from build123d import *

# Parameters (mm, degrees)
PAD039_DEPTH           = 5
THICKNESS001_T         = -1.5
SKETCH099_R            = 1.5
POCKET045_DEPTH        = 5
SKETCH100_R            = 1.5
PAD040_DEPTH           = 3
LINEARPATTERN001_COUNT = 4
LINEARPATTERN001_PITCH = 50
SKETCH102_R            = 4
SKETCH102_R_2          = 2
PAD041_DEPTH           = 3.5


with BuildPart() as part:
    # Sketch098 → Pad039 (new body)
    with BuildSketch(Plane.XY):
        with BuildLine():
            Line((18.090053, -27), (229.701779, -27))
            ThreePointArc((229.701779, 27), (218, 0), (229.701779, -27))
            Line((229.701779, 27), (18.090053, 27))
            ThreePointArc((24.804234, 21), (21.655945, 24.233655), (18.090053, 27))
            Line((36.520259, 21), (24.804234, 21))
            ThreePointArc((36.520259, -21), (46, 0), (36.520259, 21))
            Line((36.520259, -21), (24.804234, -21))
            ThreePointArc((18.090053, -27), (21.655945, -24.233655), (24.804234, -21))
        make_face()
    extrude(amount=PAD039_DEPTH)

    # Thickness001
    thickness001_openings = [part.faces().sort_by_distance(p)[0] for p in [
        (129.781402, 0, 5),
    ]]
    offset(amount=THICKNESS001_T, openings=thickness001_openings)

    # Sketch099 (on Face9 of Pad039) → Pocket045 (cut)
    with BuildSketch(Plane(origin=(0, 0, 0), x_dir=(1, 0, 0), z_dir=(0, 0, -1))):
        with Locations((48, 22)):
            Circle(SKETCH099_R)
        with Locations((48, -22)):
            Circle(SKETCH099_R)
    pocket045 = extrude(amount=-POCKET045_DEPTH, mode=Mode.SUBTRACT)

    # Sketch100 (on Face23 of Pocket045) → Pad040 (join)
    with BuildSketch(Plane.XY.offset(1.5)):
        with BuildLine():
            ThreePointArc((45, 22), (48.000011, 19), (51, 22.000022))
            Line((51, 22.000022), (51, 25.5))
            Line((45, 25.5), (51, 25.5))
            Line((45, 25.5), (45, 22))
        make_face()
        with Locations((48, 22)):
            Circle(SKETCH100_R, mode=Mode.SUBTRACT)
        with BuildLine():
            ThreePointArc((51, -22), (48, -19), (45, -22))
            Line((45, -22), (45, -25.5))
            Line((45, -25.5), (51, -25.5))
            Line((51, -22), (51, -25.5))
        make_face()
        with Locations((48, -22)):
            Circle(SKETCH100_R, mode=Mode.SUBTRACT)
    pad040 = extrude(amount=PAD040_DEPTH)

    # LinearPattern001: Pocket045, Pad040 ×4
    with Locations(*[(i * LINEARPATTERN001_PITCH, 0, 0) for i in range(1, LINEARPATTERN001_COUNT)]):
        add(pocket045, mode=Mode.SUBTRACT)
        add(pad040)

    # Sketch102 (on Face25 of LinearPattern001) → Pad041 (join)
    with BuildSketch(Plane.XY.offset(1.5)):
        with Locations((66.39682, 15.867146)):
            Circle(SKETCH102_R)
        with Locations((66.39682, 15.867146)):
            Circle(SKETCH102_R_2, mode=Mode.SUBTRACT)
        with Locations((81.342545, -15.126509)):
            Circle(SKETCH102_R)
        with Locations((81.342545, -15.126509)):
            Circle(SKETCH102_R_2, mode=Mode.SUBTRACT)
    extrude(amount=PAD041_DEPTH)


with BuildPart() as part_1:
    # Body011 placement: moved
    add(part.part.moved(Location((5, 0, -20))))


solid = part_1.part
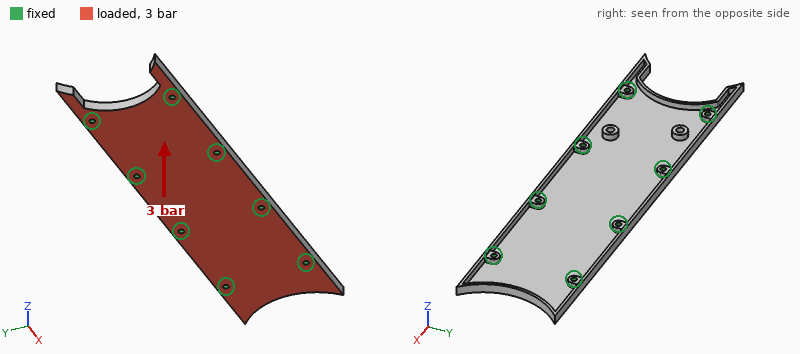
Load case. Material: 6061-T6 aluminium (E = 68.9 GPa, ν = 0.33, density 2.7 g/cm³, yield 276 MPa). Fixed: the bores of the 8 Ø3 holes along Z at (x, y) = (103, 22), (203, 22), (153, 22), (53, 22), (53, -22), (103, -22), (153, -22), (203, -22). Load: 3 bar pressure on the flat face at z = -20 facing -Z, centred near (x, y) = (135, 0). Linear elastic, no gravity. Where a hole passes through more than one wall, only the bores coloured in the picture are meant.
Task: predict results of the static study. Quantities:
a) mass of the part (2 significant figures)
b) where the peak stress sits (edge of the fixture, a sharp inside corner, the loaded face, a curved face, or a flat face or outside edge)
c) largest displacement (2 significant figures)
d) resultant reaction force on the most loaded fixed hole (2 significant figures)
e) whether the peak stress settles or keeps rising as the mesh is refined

50 g
edge of the fixture
0.31 mm
440 N
keeps rising
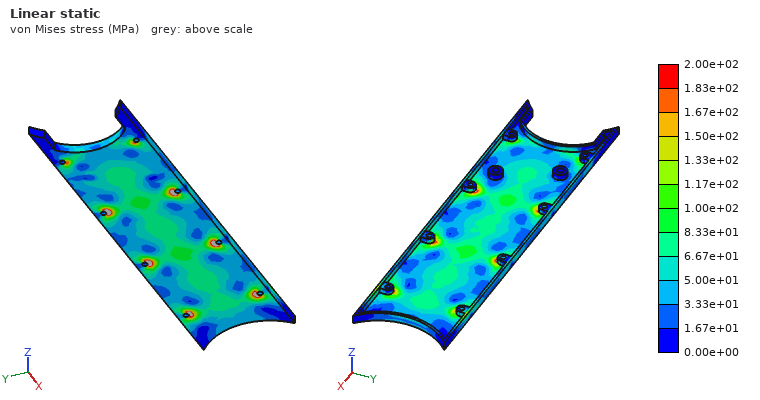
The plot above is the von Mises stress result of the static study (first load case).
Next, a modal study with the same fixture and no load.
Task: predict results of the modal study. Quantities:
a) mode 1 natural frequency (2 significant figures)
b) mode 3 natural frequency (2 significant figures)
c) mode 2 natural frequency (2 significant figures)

2700 Hz
3000 Hz
3000 Hz
